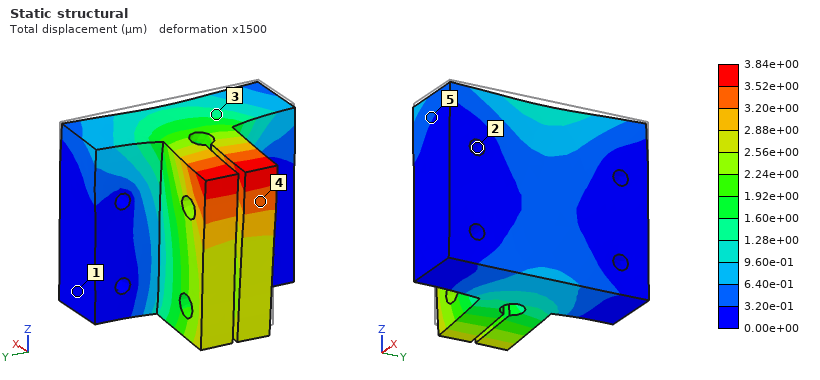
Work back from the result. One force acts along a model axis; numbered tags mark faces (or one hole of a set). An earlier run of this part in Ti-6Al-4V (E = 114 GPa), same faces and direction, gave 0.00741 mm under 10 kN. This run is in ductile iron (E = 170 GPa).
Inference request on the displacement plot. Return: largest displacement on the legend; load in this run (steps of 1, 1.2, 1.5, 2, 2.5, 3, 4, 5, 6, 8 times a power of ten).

3.84e+00 µm
8 kN
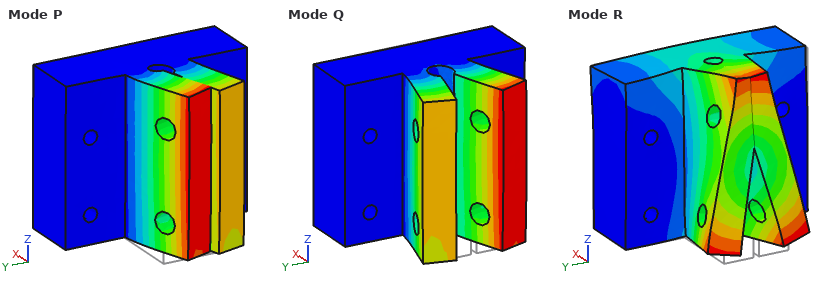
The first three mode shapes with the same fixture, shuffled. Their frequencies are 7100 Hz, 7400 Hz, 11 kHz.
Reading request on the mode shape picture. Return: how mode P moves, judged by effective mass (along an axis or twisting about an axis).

along Y
